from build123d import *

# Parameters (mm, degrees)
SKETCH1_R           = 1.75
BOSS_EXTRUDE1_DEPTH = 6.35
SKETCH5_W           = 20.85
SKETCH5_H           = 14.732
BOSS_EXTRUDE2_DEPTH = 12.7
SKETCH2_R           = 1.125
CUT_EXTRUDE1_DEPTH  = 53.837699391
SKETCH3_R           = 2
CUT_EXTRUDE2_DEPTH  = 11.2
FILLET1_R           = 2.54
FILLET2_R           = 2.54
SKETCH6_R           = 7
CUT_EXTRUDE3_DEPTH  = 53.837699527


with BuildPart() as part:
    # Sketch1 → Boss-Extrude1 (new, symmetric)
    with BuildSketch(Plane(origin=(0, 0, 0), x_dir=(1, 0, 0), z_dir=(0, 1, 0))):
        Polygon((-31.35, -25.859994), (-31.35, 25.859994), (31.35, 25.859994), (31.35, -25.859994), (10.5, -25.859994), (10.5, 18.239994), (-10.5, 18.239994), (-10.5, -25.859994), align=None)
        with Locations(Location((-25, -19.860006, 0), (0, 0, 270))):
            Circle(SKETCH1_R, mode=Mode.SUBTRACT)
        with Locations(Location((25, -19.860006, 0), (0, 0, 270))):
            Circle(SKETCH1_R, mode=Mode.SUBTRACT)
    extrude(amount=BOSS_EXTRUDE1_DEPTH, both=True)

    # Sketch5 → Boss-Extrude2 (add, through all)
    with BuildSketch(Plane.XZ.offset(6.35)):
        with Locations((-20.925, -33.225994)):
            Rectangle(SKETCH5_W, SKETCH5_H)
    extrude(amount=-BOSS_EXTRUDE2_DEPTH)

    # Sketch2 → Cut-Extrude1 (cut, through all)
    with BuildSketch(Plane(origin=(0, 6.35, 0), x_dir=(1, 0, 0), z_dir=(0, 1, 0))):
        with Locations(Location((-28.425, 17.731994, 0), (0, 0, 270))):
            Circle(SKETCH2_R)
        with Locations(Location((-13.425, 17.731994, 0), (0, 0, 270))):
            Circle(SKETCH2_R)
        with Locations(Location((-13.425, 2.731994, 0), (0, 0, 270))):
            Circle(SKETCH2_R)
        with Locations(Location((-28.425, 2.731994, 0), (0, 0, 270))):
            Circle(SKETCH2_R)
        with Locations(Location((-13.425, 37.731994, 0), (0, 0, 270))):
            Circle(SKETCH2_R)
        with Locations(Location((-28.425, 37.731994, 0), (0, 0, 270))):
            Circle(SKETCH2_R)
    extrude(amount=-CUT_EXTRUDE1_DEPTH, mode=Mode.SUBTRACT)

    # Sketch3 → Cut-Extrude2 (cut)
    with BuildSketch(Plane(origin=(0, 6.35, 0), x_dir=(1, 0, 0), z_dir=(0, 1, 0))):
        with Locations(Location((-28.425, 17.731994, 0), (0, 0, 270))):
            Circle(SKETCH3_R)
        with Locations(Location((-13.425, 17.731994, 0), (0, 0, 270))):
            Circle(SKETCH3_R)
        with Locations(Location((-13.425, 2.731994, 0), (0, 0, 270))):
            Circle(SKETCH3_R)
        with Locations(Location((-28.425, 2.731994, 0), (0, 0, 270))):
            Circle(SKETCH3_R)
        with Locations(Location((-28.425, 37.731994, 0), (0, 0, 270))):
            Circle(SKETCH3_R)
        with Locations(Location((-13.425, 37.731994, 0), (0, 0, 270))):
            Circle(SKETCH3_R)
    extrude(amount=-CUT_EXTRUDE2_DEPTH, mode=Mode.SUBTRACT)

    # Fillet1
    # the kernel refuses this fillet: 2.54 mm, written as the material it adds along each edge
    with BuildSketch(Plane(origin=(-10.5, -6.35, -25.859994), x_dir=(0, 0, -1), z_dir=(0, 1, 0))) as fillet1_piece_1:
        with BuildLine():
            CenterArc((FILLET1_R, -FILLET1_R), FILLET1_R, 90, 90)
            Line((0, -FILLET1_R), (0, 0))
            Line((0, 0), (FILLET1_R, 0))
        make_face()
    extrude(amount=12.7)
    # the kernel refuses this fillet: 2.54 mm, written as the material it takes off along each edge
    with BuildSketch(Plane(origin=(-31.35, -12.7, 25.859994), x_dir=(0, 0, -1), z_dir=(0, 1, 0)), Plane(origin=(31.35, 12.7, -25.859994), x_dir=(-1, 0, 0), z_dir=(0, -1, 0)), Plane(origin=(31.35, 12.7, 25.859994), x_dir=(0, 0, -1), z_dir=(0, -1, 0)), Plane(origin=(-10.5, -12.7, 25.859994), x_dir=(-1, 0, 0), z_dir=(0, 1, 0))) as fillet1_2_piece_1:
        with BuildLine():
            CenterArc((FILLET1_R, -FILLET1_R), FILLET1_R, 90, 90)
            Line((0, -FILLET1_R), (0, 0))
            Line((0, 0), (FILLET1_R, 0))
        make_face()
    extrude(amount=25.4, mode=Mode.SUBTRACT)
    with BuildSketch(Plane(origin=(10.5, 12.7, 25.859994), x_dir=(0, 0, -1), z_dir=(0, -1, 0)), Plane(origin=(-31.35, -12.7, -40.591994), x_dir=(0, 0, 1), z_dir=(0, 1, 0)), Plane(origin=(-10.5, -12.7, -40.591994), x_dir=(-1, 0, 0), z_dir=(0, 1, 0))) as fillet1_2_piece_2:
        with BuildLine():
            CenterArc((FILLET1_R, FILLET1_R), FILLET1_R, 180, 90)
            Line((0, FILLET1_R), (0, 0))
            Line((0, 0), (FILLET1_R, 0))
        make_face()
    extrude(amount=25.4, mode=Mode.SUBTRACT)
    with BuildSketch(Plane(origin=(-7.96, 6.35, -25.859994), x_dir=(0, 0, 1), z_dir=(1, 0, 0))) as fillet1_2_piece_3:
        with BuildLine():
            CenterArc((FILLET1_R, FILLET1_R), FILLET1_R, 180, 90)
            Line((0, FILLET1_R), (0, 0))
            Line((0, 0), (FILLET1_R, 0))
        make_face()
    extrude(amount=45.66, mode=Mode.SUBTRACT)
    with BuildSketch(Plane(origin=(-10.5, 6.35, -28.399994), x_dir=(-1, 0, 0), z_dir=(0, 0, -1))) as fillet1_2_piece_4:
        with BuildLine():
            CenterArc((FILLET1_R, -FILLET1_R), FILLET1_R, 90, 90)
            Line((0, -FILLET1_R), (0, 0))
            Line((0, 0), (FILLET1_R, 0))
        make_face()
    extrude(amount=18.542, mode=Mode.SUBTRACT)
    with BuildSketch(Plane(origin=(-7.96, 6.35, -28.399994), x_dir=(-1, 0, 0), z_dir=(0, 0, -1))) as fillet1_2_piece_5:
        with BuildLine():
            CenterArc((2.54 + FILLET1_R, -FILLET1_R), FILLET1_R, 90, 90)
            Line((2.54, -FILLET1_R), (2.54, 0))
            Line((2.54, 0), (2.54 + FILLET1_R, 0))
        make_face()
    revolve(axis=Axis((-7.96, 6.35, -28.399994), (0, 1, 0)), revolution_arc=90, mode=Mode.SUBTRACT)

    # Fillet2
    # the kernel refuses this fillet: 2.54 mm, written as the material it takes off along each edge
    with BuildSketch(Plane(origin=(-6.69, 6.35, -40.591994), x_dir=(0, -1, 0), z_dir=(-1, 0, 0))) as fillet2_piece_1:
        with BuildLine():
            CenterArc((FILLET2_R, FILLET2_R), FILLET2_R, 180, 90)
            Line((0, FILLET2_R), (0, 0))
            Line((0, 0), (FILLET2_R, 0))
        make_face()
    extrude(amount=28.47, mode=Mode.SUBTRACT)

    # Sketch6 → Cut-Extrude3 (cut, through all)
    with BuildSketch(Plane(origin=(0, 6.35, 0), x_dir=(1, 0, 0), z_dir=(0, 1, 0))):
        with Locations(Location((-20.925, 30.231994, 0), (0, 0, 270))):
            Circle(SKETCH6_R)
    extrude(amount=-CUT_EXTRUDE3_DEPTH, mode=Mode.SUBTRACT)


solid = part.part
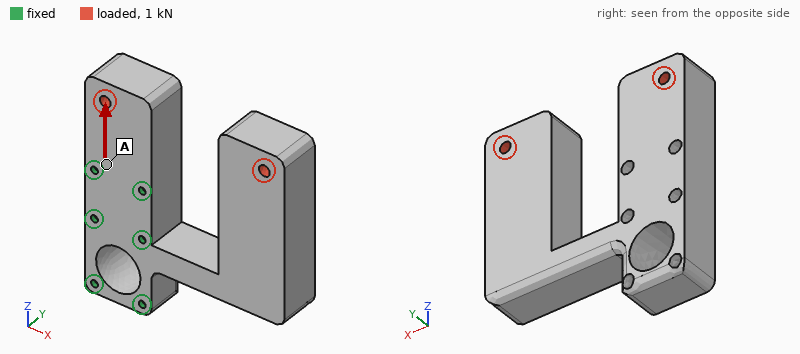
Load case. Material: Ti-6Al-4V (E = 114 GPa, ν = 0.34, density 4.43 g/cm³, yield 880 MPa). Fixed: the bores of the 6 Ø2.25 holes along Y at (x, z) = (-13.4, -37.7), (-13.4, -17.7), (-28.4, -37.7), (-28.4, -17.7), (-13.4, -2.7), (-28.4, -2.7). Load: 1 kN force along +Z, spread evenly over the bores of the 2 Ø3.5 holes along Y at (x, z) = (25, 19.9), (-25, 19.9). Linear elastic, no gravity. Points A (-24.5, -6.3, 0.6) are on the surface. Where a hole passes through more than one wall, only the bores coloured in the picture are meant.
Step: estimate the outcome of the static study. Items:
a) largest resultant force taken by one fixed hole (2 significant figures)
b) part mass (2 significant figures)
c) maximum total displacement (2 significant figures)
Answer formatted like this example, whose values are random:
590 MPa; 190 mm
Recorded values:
630 N; 130 g; 0.41 mm
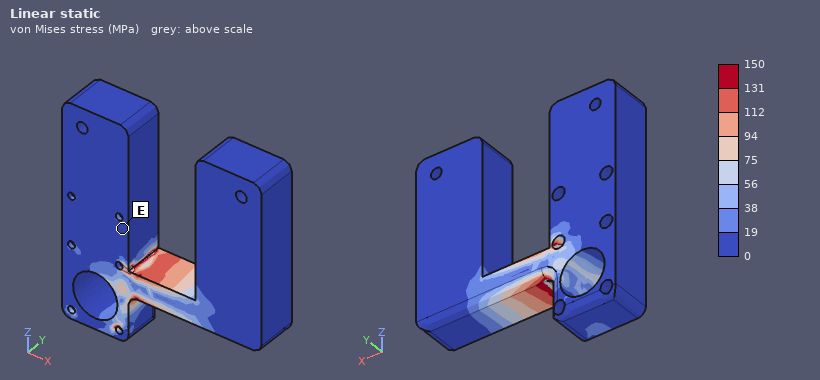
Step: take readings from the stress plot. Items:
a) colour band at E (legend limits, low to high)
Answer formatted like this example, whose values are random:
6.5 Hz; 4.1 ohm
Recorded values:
0 to 19 MPa
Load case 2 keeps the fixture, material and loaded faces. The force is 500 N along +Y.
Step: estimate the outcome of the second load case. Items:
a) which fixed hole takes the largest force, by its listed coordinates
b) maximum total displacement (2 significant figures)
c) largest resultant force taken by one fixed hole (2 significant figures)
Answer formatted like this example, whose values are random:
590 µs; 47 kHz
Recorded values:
(-13.4, -17.7); 0.33 mm; 630 N
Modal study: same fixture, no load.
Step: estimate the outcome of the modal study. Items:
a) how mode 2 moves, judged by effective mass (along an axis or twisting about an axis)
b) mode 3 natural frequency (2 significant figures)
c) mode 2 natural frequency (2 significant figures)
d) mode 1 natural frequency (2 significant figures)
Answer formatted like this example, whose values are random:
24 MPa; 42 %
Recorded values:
along Y; 2800 Hz; 920 Hz; 790 Hz
